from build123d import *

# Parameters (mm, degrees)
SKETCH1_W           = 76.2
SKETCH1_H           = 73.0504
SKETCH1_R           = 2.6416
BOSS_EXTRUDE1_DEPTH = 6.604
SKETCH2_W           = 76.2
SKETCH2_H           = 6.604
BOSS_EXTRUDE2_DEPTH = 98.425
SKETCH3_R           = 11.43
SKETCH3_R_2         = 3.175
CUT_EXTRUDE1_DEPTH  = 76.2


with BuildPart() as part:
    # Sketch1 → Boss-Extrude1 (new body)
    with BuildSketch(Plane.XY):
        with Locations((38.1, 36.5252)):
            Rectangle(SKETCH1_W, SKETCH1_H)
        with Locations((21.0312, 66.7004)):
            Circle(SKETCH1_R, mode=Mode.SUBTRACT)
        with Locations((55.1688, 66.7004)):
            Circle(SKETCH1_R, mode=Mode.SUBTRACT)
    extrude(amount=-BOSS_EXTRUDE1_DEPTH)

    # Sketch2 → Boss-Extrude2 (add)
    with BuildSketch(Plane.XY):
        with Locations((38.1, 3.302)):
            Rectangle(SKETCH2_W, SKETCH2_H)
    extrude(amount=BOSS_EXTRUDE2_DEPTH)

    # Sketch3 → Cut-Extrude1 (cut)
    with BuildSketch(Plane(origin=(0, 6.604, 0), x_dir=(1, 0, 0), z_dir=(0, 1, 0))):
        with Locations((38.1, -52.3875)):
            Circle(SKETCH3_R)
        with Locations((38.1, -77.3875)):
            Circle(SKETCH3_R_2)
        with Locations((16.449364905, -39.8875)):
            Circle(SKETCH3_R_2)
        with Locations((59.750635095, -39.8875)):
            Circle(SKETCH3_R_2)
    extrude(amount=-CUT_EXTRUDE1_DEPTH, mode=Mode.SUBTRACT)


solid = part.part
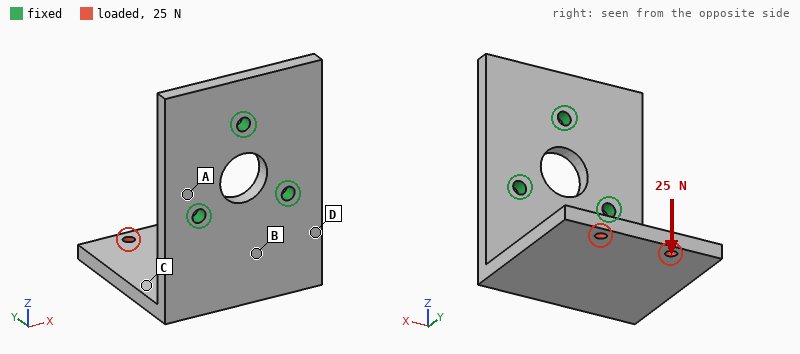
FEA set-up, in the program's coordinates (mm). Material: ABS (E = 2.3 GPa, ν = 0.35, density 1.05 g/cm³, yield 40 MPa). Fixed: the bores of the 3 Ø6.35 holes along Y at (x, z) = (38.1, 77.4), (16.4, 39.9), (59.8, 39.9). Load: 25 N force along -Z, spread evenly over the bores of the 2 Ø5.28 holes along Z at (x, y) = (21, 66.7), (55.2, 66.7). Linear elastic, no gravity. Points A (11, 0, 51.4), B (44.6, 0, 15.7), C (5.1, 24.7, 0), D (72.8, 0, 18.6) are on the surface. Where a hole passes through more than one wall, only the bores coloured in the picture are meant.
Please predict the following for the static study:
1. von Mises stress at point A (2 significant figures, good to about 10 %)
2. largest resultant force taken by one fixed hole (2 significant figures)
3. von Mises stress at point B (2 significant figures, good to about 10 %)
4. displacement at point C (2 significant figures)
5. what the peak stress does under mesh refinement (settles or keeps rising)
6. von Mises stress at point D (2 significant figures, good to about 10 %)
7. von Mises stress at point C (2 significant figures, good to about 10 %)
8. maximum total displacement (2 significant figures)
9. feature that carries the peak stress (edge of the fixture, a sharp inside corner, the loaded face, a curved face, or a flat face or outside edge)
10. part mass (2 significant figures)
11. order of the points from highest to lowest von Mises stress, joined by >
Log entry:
0.45 MPa
14 N
2.4 MPa
0.48 mm
keeps rising
2.9 MPa
1.8 MPa
1.6 mm
edge of the fixture
87 g
D > B > C > A
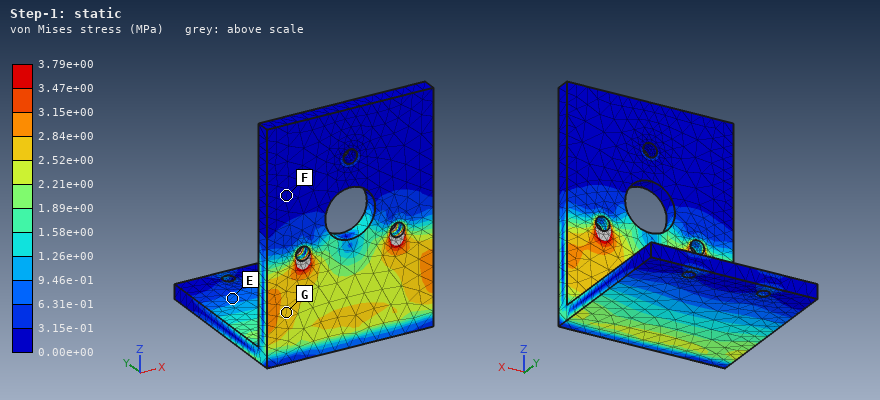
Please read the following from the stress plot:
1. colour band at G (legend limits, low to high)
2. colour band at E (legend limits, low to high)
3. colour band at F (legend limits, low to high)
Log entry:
2.52e+00 to 2.84e+00 MPa
6.31e-01 to 9.46e-01 MPa
0.00e+00 to 3.15e-01 MPa
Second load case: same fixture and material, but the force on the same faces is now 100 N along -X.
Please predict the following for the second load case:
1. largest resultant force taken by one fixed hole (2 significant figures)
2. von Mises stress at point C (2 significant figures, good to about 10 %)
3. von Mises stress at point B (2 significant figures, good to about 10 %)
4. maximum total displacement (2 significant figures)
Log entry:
160 N
2.9 MPa
5.5 MPa
1.7 mm
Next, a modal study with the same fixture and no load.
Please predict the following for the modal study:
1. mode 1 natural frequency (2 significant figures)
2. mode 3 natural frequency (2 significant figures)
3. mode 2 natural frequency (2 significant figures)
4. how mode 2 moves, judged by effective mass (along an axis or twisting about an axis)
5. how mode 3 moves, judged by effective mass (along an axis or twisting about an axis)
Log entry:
160 Hz
490 Hz
300 Hz
along X
along Y
